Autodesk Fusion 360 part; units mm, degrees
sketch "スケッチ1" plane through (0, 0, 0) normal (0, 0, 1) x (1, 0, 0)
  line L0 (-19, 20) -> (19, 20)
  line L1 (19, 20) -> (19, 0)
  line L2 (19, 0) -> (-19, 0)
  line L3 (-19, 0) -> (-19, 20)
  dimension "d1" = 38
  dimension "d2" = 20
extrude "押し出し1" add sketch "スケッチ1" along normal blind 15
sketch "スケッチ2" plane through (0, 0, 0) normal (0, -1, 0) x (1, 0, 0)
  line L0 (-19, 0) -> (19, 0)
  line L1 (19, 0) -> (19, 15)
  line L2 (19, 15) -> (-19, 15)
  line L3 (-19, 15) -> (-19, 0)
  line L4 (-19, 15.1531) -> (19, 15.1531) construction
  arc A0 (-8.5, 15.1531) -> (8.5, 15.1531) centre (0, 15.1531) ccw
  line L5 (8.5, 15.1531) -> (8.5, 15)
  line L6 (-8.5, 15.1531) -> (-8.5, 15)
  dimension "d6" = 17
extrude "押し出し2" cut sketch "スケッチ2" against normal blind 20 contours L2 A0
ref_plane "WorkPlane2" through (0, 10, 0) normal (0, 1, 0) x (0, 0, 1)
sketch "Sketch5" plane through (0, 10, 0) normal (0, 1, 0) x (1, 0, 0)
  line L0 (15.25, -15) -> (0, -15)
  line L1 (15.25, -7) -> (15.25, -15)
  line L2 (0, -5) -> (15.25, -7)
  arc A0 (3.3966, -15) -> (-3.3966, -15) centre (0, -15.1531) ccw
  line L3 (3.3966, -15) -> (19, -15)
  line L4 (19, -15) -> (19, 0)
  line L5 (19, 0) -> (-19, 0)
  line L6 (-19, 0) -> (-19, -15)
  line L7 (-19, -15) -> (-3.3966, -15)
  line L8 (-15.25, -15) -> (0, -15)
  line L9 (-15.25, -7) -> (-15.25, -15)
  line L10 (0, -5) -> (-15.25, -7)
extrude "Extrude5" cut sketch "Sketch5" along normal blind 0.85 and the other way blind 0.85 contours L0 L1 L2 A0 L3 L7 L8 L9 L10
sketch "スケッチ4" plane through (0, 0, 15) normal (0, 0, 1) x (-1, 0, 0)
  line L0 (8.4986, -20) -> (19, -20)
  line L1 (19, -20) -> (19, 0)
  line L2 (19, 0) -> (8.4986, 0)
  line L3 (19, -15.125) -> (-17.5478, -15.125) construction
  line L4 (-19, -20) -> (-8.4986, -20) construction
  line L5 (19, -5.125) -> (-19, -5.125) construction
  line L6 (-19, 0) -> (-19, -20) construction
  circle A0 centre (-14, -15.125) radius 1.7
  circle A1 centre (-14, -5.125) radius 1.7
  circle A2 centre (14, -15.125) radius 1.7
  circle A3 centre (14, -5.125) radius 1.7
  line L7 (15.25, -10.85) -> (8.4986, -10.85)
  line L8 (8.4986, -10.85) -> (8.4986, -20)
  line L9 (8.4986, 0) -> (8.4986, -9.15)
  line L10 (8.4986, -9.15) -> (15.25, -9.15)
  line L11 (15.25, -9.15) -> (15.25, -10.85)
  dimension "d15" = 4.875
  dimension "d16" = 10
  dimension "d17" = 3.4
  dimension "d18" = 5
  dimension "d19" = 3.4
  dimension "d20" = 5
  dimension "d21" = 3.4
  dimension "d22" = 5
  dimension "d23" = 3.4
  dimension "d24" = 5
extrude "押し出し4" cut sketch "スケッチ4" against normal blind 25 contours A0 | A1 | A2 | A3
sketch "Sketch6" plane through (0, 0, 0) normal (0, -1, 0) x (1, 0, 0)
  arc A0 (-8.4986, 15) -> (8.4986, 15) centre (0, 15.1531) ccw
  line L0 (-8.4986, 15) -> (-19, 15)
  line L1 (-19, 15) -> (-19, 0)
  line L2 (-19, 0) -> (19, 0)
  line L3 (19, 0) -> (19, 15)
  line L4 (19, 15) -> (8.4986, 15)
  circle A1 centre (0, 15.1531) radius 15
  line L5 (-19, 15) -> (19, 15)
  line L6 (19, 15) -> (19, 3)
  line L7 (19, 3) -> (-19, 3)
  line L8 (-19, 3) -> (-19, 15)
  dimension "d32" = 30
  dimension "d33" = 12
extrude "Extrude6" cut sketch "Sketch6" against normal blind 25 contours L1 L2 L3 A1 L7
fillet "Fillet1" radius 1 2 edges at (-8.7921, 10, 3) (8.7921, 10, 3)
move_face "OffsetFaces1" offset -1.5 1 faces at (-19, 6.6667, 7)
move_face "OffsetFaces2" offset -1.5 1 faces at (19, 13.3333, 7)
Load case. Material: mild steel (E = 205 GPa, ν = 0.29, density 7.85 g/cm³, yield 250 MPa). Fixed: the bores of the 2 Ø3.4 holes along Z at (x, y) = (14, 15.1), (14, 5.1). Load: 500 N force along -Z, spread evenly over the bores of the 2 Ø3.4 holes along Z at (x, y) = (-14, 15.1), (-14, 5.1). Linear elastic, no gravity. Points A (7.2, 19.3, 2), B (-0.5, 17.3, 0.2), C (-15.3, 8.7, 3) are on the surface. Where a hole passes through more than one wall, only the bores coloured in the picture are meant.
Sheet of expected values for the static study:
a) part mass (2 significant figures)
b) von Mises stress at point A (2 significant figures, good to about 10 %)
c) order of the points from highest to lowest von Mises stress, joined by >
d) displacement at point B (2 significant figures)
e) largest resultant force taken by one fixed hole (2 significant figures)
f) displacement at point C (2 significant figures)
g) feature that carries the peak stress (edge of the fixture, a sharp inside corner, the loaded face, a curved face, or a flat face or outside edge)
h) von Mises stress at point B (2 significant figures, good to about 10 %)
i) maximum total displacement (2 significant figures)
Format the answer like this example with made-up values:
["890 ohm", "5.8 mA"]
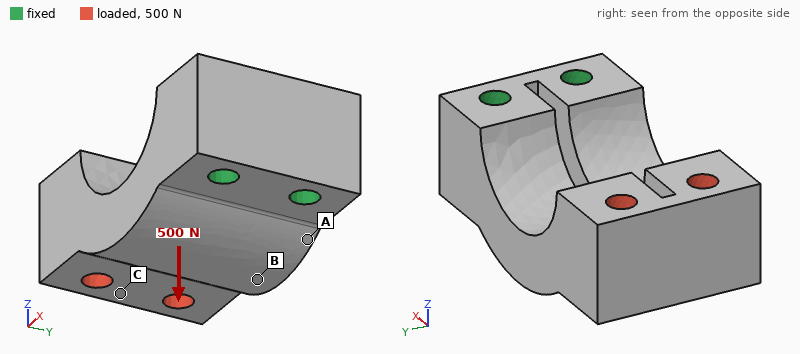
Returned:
["48 g", "60 MPa", "A > B > C", "9.8 µm", "280 N", "31 µm", "a curved face", "42 MPa", "39 µm"]
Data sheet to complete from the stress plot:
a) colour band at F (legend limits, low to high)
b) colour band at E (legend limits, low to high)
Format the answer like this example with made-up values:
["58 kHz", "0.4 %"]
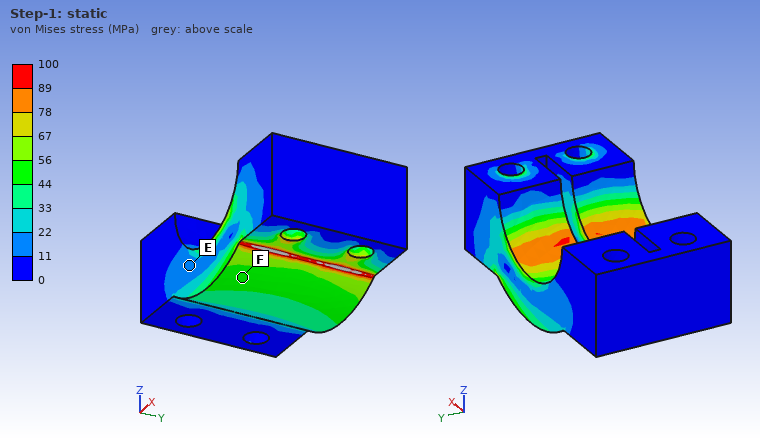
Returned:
["44 to 56 MPa", "11 to 22 MPa"]
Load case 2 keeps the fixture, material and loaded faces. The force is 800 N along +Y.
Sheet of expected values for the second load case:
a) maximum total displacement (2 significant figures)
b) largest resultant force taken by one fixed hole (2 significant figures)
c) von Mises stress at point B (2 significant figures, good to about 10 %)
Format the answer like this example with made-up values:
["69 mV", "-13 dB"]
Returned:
["23 µm", "1.6 kN", "18 MPa"]
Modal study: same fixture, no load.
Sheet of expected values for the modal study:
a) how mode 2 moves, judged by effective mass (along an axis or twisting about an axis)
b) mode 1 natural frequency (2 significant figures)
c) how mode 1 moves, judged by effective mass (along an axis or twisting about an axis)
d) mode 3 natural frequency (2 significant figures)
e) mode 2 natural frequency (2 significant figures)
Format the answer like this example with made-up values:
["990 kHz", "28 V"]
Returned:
["along Y", "5100 Hz", "along Z", "16 kHz", "8200 Hz"]
